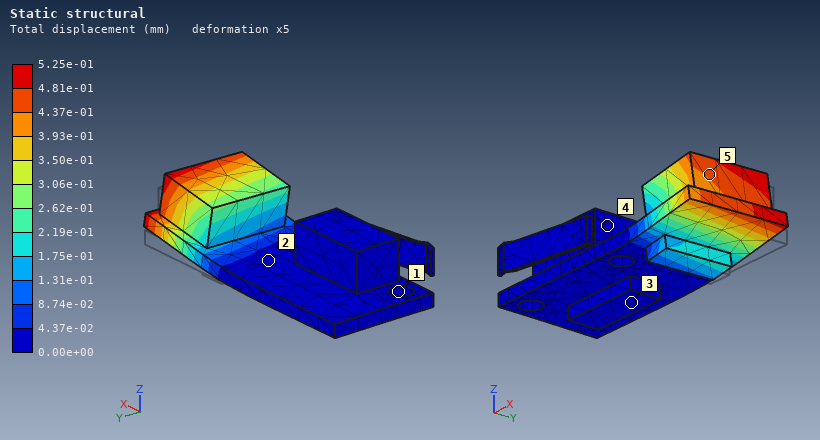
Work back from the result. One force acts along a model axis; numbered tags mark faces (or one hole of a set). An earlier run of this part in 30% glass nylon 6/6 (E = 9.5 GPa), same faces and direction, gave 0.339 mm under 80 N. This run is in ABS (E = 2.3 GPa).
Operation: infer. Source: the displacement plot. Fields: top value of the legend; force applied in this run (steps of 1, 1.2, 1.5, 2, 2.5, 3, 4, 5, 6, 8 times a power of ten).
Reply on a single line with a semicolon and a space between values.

5.25e-01 mm; 30 N
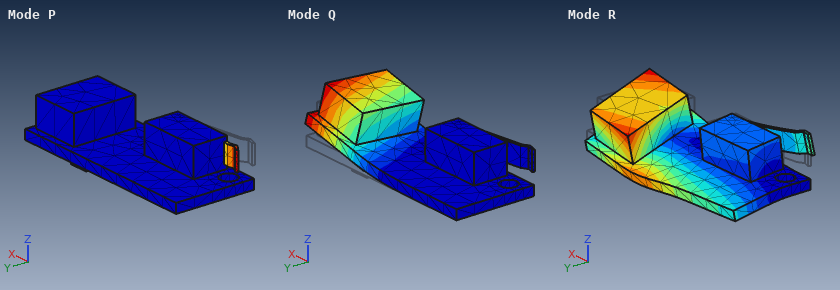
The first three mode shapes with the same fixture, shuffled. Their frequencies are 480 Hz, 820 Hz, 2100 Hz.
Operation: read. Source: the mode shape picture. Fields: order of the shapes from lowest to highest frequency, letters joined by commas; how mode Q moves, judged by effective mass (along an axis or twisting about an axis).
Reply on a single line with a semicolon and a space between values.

P, Q, R; along Z
